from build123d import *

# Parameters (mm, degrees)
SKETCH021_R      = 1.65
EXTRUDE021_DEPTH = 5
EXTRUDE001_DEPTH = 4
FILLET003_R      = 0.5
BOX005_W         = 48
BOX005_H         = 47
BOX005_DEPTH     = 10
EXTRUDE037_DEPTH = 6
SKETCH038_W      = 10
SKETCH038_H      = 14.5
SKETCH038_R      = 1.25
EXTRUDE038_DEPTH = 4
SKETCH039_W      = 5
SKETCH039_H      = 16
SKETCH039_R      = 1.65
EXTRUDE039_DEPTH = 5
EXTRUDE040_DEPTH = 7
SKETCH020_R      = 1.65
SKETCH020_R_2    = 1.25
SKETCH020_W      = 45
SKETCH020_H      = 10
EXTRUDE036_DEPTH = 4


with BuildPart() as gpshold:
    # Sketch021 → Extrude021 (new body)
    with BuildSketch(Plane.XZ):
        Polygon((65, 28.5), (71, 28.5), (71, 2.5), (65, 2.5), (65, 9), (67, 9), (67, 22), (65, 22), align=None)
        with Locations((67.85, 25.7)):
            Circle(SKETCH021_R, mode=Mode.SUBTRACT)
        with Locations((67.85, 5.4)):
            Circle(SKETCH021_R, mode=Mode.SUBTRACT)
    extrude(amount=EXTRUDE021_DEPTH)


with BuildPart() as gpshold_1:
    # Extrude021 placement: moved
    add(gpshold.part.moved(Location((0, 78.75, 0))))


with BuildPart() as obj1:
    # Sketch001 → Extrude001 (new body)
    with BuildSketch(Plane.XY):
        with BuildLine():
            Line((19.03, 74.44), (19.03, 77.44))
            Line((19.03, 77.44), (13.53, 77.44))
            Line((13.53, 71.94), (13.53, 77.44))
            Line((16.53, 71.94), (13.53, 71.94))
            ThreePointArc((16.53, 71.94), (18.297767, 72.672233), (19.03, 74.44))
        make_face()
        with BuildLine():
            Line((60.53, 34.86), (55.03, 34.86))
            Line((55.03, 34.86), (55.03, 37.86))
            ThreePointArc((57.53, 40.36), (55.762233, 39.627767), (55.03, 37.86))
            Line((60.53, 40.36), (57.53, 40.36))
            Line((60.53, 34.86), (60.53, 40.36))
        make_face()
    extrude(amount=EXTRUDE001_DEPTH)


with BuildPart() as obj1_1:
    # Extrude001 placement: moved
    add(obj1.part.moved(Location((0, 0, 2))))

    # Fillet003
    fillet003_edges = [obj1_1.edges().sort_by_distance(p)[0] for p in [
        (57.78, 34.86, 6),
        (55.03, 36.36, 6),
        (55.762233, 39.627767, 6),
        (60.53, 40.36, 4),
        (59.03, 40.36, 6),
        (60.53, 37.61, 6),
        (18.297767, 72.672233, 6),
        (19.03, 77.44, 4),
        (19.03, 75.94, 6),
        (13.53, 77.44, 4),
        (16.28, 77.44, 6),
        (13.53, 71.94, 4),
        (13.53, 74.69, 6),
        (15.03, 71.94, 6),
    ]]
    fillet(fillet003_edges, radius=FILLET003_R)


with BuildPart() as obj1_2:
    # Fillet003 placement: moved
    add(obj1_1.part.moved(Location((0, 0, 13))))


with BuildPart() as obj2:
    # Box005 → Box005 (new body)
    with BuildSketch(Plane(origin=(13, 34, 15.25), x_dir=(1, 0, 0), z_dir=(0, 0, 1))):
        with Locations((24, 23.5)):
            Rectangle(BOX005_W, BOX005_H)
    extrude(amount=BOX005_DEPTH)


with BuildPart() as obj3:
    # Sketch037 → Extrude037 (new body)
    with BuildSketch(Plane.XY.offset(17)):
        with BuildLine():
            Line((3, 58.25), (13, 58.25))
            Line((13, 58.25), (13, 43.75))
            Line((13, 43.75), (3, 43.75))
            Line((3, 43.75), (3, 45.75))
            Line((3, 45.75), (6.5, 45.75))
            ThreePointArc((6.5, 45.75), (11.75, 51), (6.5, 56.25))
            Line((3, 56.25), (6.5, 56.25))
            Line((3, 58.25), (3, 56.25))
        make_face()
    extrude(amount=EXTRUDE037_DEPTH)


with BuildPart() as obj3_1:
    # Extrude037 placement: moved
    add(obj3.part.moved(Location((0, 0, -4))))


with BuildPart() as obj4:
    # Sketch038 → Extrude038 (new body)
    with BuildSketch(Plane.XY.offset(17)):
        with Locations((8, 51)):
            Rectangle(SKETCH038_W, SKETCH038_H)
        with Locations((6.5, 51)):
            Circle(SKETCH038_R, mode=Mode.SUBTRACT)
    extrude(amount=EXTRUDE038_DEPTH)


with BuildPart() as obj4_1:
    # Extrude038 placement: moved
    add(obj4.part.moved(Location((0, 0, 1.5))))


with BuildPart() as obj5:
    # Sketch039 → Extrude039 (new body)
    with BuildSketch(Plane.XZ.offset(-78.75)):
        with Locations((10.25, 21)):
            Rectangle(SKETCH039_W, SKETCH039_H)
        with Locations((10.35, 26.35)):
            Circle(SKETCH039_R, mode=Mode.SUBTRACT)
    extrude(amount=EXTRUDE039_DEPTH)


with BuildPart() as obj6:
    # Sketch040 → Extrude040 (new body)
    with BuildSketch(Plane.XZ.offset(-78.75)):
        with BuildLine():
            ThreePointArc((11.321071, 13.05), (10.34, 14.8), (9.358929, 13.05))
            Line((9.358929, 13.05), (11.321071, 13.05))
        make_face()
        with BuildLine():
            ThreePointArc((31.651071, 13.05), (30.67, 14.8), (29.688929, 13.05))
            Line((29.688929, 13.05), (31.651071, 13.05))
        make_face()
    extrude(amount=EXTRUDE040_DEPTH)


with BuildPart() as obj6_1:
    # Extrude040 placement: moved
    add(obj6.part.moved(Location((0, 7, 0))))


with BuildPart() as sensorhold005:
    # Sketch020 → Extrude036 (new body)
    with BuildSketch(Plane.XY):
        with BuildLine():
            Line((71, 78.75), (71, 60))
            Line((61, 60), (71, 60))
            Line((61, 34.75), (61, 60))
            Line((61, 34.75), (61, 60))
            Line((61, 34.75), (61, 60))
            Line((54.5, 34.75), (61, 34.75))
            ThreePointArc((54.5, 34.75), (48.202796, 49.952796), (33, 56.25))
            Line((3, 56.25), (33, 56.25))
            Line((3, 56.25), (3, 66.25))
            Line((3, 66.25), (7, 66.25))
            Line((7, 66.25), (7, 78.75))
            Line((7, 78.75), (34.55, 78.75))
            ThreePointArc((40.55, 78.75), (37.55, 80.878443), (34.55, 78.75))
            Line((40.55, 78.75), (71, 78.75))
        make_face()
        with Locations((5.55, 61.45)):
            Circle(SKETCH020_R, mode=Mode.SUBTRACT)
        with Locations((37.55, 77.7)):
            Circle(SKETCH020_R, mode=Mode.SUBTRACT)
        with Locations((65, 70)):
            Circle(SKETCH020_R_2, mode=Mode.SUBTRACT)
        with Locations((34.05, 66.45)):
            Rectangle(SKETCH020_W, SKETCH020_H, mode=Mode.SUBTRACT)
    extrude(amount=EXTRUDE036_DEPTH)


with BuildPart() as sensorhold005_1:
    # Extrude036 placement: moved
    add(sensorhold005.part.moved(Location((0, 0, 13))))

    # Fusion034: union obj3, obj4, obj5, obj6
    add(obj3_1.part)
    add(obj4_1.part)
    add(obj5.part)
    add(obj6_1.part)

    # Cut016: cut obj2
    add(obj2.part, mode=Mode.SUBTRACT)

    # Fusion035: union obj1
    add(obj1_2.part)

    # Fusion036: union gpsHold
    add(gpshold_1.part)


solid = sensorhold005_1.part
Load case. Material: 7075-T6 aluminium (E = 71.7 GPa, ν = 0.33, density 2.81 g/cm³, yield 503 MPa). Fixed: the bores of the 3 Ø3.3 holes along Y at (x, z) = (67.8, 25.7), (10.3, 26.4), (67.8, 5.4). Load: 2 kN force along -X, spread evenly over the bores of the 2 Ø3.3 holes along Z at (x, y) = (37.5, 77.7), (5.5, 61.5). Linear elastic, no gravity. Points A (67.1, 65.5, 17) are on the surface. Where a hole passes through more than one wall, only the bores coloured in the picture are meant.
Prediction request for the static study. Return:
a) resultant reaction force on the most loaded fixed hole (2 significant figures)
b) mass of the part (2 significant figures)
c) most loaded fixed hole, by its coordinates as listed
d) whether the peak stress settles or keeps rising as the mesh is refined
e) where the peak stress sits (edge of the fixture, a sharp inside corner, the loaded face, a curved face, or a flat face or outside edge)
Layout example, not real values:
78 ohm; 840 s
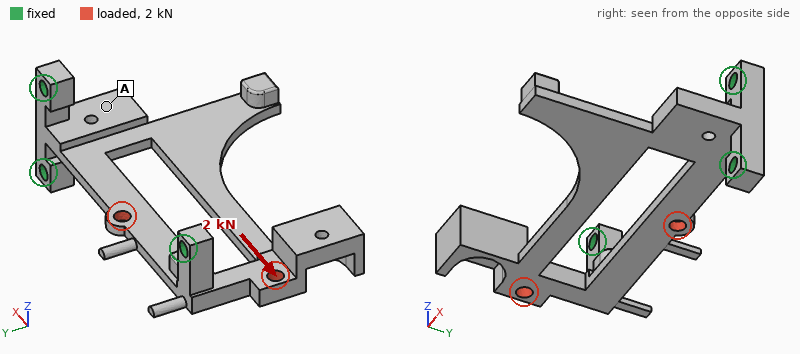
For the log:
900 N; 15 g; (67.8, 5.4); keeps rising; edge of the fixture
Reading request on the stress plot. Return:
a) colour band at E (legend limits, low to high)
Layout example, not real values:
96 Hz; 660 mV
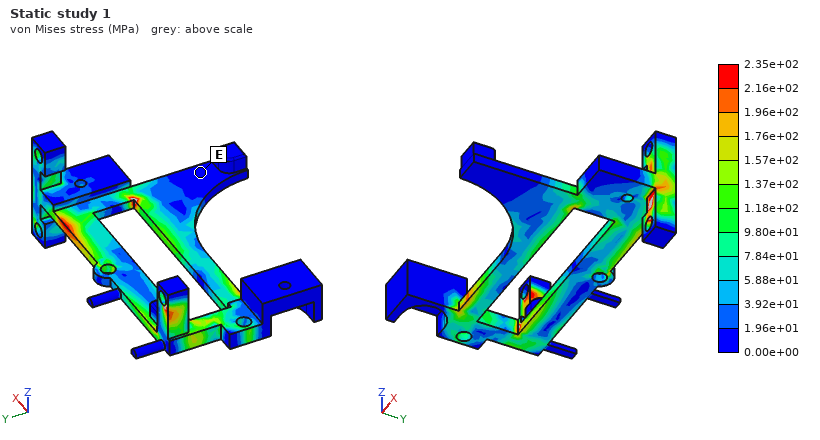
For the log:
0.00e+00 to 1.96e+01 MPa
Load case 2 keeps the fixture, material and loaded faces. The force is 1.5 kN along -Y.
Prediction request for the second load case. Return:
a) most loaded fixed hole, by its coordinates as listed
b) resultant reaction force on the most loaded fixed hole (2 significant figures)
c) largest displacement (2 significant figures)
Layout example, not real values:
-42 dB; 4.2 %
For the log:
(10.3, 26.4); 1.3 kN; 0.66 mm
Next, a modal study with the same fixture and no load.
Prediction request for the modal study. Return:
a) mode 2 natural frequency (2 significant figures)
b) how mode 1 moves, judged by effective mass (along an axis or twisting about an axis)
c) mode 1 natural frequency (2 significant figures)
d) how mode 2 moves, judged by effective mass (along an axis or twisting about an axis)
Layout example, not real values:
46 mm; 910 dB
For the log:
1600 Hz; along Z; 1300 Hz; twisting about Y
